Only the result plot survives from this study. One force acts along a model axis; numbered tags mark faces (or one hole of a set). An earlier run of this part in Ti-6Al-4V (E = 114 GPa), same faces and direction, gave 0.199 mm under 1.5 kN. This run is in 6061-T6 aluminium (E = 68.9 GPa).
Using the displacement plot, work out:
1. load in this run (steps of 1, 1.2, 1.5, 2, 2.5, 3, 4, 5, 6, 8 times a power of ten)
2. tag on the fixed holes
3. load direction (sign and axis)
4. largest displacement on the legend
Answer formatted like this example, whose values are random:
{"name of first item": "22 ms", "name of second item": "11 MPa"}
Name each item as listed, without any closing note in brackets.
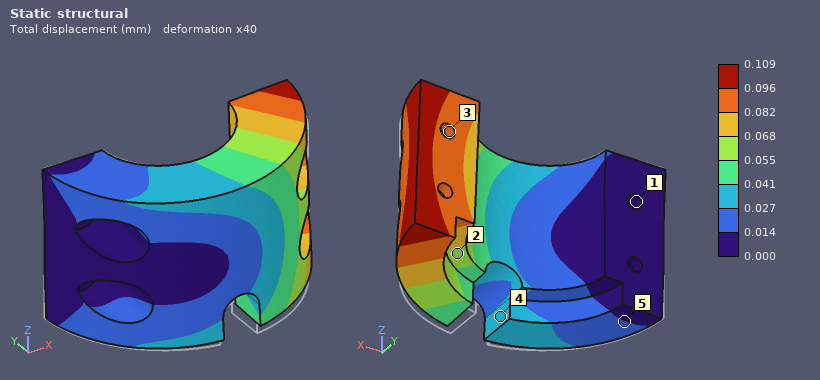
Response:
{"load in this run": "500 N", "tag on the fixed holes": "1", "load direction": "+Z", "largest displacement on the legend": "0.109 mm"}
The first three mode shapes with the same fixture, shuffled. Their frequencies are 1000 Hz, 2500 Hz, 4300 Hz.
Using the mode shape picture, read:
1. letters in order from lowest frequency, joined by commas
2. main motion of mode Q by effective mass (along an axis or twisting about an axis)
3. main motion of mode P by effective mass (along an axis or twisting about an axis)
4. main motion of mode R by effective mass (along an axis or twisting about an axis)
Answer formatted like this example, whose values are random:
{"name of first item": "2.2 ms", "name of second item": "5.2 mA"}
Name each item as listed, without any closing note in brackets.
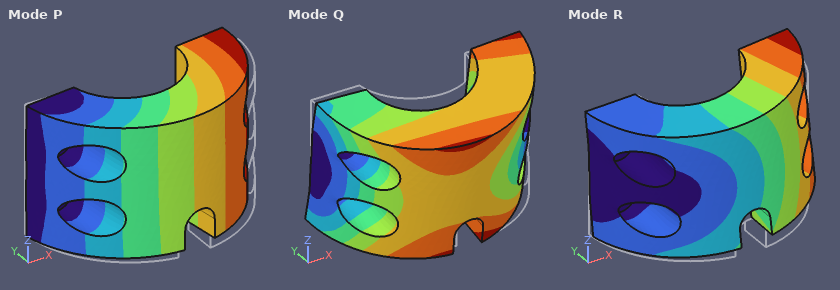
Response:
{"letters in order from lowest frequency, joined by commas": "P, R, Q", "main motion of mode Q by effective mass": "along Z", "main motion of mode P by effective mass": "along Y", "main motion of mode R by effective mass": "along Z"}
